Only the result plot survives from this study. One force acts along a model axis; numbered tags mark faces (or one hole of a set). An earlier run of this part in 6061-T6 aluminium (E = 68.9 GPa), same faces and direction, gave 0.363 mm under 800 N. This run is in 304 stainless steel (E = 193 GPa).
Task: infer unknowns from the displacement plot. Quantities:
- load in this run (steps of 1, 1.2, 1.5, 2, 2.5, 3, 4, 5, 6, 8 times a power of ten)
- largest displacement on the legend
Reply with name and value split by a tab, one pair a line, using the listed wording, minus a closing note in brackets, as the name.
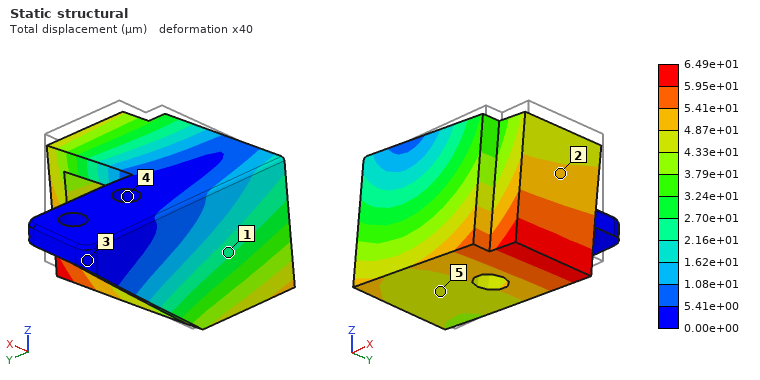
load in this run	400 N
largest displacement on the legend	6.49e+01 µm
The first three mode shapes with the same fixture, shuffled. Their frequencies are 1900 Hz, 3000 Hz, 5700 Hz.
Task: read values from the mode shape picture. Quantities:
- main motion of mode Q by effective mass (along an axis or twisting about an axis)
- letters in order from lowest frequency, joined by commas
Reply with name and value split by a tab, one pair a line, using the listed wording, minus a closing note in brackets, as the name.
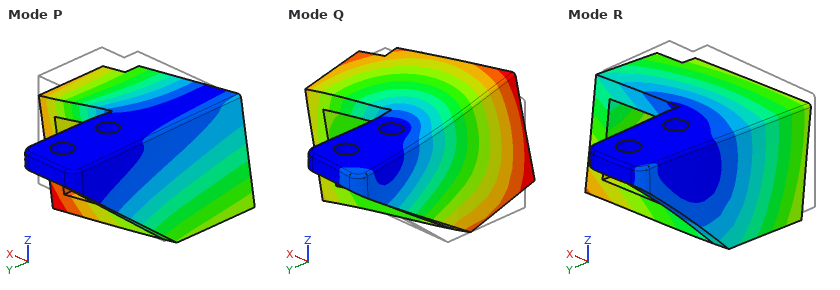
main motion of mode Q by effective mass	along Z
letters in order from lowest frequency, joined by commas	P, R, Q
